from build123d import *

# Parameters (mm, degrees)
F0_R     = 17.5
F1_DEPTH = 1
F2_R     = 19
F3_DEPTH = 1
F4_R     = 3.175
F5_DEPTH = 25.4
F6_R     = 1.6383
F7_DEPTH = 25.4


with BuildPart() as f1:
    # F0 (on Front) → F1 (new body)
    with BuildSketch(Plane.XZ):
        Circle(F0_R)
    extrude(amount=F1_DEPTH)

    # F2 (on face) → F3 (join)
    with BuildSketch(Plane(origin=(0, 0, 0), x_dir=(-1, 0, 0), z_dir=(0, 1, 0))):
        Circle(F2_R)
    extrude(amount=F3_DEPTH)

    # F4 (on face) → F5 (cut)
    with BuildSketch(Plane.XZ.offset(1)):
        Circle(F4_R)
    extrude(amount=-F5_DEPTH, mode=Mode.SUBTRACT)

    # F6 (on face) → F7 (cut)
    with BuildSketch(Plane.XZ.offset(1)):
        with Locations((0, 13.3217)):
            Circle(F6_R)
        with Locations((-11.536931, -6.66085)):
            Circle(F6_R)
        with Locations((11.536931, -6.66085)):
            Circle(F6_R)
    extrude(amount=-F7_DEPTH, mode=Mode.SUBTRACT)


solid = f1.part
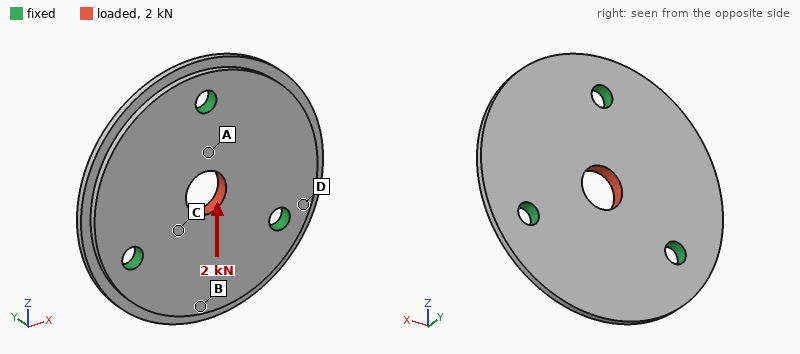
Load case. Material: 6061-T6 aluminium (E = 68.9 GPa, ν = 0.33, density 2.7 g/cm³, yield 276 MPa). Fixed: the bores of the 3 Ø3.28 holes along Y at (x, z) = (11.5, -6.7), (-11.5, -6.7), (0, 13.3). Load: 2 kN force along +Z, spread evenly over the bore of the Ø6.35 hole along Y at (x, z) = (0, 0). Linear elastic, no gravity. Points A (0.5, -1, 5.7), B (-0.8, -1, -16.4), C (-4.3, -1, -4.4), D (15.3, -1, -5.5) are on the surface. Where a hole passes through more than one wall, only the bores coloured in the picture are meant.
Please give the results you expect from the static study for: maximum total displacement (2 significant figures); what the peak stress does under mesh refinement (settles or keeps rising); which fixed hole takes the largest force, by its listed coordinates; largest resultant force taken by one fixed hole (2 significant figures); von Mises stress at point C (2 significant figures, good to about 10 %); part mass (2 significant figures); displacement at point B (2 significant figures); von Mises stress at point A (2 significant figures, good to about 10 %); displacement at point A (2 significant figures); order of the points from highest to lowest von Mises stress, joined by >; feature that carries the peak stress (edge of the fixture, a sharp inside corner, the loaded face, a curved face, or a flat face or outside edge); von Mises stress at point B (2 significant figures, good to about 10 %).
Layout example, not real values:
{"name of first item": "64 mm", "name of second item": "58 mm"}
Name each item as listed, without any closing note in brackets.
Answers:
{"maximum total displacement": "9.6 µm", "what the peak stress does under mesh refinement": "keeps rising", "which fixed hole takes the largest force, by its listed coordinates": "(0, 13.3)", "largest resultant force taken by one fixed hole": "720 N", "von Mises stress at point C": "32 MPa", "part mass": "5.4 g", "displacement at point B": "5.1 µm", "von Mises stress at point A": "53 MPa", "displacement at point A": "4.7 µm", "order of the points from highest to lowest von Mises stress, joined by >": "A > C > B > D", "feature that carries the peak stress": "edge of the fixture", "von Mises stress at point B": "19 MPa"}
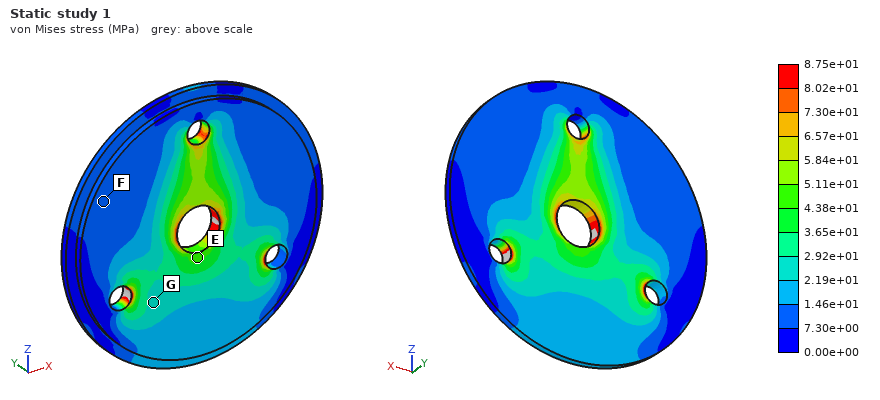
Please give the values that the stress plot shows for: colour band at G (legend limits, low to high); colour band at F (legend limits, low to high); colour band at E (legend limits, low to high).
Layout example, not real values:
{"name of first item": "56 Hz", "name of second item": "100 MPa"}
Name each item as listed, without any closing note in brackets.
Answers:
{"colour band at G": "2.19e+01 to 2.92e+01 MPa", "colour band at F": "7.30e+00 to 1.46e+01 MPa", "colour band at E": "4.38e+01 to 5.11e+01 MPa"}
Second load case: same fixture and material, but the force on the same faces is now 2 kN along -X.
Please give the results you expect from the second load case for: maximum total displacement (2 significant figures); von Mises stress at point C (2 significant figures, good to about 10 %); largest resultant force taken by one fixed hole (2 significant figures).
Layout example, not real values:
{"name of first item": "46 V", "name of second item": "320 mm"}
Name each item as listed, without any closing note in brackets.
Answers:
{"maximum total displacement": "9.3 µm", "von Mises stress at point C": "42 MPa", "largest resultant force taken by one fixed hole": "700 N"}
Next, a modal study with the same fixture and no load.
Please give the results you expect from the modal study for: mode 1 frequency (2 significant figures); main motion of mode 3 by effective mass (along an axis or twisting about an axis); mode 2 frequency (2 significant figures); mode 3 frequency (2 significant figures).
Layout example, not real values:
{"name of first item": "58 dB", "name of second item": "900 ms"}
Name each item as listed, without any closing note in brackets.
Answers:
{"mode 1 frequency": "12 kHz", "main motion of mode 3 by effective mass": "along Y", "mode 2 frequency": "12 kHz", "mode 3 frequency": "13 kHz"}
